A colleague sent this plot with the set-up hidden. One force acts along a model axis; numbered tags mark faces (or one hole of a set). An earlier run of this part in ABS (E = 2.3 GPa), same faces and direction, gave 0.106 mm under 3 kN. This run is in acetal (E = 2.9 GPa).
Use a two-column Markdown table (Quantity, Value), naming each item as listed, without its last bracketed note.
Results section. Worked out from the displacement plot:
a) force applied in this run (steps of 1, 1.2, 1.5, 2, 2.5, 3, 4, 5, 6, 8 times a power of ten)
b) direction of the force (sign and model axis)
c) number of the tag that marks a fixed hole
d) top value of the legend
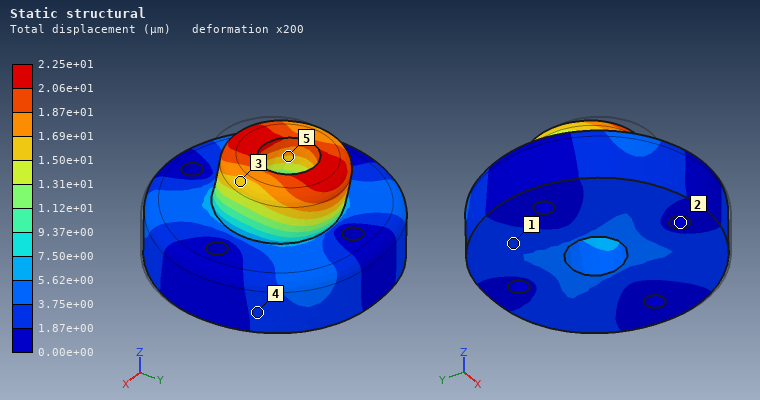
| Quantity | Value |
|---|---|
| force applied in this run | 800 N |
| direction of the force | +Y |
| number of the tag that marks a fixed hole | 2 |
| top value of the legend | 2.25e+01 µm |
